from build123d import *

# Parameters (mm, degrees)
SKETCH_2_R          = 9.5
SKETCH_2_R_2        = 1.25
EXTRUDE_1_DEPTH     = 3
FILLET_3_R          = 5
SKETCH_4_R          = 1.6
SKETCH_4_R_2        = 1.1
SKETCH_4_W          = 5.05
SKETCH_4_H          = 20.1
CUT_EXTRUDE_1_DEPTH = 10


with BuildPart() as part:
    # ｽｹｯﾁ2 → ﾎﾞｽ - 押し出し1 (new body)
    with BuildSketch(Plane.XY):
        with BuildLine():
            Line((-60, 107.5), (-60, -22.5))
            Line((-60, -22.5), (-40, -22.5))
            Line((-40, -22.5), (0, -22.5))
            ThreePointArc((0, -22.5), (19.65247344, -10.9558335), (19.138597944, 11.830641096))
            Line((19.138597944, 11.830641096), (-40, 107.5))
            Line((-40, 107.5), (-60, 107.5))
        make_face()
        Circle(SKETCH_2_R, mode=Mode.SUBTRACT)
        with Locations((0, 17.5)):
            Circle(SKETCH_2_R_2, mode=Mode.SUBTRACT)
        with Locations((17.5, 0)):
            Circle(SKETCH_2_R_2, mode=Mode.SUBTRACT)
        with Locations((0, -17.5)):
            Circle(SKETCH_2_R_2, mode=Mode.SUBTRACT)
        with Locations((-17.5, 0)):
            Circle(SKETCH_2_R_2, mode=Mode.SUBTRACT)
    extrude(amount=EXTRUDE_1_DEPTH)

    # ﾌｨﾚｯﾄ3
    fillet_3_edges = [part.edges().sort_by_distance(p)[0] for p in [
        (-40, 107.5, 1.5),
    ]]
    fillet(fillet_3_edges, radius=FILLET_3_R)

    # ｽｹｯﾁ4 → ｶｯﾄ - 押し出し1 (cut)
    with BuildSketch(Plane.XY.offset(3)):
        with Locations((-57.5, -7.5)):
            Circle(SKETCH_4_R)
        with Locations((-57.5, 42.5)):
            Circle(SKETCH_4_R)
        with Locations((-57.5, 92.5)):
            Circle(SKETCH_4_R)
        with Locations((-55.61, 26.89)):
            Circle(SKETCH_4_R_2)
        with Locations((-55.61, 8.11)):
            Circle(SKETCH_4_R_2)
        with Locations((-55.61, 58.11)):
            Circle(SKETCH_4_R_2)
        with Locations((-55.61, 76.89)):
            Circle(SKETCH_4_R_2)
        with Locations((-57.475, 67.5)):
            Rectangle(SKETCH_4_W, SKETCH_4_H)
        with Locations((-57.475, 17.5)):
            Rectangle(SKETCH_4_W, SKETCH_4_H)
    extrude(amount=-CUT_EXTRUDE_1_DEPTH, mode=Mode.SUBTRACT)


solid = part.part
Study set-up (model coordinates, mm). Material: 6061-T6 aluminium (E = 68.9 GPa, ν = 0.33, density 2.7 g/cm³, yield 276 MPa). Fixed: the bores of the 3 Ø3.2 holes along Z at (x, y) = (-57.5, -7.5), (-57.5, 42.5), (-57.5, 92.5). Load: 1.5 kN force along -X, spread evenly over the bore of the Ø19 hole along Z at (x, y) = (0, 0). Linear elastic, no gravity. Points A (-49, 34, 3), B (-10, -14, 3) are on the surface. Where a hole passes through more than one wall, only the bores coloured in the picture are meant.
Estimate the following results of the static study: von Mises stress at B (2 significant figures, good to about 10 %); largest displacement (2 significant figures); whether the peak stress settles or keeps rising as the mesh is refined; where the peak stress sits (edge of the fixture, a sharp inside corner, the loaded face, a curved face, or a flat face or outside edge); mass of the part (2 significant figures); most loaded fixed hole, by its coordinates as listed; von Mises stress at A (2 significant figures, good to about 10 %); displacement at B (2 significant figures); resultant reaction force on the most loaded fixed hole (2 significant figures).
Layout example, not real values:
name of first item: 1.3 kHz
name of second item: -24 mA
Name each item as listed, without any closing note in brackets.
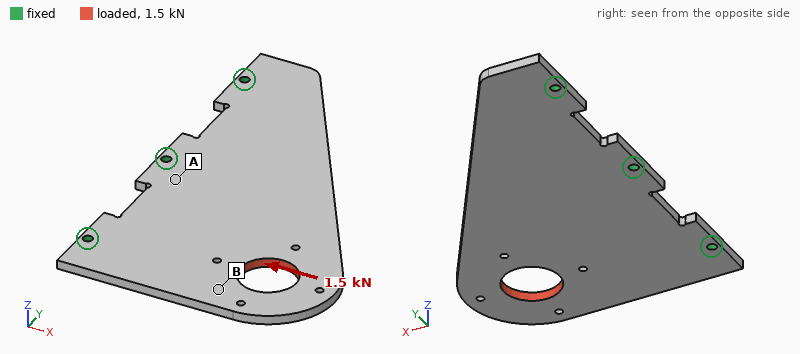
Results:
von Mises stress at B: 15 MPa
largest displacement: 21 µm
whether the peak stress settles or keeps rising as the mesh is refined: keeps rising
where the peak stress sits: edge of the fixture
mass of the part: 56 g
most loaded fixed hole, by its coordinates as listed: (-57.5, -7.5)
von Mises stress at A: 6.8 MPa
displacement at B: 16 µm
resultant reaction force on the most loaded fixed hole: 1.2 kN
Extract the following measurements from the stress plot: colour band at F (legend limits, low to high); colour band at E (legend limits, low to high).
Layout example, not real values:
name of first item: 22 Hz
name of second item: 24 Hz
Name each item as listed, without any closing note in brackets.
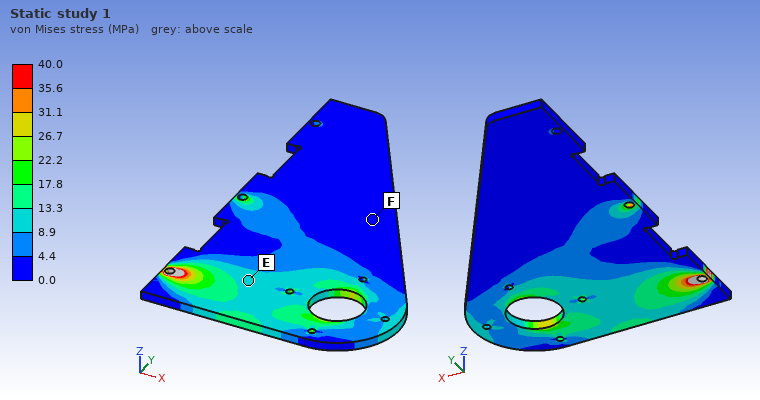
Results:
colour band at F: 0.0 to 4.4 MPa
colour band at E: 8.9 to 13.3 MPa
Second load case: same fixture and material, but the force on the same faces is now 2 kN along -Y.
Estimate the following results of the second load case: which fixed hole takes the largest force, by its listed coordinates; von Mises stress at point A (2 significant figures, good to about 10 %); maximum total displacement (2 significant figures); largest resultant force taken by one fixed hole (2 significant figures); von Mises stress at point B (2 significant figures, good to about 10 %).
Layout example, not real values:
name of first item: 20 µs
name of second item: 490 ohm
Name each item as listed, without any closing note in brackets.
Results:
which fixed hole takes the largest force, by its listed coordinates: (-57.5, -7.5)
von Mises stress at point A: 14 MPa
maximum total displacement: 52 µm
largest resultant force taken by one fixed hole: 1.4 kN
von Mises stress at point B: 17 MPa
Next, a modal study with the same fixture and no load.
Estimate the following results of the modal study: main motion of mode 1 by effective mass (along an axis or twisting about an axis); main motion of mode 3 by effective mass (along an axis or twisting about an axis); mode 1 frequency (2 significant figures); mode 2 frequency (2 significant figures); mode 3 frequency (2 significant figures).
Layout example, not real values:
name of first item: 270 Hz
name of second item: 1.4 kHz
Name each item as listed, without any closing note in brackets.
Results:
main motion of mode 1 by effective mass: along Z
main motion of mode 3 by effective mass: along Z
mode 1 frequency: 470 Hz
mode 2 frequency: 1200 Hz
mode 3 frequency: 2300 Hz
